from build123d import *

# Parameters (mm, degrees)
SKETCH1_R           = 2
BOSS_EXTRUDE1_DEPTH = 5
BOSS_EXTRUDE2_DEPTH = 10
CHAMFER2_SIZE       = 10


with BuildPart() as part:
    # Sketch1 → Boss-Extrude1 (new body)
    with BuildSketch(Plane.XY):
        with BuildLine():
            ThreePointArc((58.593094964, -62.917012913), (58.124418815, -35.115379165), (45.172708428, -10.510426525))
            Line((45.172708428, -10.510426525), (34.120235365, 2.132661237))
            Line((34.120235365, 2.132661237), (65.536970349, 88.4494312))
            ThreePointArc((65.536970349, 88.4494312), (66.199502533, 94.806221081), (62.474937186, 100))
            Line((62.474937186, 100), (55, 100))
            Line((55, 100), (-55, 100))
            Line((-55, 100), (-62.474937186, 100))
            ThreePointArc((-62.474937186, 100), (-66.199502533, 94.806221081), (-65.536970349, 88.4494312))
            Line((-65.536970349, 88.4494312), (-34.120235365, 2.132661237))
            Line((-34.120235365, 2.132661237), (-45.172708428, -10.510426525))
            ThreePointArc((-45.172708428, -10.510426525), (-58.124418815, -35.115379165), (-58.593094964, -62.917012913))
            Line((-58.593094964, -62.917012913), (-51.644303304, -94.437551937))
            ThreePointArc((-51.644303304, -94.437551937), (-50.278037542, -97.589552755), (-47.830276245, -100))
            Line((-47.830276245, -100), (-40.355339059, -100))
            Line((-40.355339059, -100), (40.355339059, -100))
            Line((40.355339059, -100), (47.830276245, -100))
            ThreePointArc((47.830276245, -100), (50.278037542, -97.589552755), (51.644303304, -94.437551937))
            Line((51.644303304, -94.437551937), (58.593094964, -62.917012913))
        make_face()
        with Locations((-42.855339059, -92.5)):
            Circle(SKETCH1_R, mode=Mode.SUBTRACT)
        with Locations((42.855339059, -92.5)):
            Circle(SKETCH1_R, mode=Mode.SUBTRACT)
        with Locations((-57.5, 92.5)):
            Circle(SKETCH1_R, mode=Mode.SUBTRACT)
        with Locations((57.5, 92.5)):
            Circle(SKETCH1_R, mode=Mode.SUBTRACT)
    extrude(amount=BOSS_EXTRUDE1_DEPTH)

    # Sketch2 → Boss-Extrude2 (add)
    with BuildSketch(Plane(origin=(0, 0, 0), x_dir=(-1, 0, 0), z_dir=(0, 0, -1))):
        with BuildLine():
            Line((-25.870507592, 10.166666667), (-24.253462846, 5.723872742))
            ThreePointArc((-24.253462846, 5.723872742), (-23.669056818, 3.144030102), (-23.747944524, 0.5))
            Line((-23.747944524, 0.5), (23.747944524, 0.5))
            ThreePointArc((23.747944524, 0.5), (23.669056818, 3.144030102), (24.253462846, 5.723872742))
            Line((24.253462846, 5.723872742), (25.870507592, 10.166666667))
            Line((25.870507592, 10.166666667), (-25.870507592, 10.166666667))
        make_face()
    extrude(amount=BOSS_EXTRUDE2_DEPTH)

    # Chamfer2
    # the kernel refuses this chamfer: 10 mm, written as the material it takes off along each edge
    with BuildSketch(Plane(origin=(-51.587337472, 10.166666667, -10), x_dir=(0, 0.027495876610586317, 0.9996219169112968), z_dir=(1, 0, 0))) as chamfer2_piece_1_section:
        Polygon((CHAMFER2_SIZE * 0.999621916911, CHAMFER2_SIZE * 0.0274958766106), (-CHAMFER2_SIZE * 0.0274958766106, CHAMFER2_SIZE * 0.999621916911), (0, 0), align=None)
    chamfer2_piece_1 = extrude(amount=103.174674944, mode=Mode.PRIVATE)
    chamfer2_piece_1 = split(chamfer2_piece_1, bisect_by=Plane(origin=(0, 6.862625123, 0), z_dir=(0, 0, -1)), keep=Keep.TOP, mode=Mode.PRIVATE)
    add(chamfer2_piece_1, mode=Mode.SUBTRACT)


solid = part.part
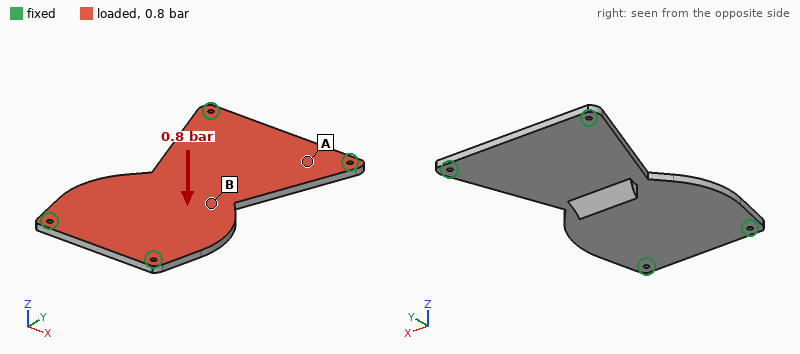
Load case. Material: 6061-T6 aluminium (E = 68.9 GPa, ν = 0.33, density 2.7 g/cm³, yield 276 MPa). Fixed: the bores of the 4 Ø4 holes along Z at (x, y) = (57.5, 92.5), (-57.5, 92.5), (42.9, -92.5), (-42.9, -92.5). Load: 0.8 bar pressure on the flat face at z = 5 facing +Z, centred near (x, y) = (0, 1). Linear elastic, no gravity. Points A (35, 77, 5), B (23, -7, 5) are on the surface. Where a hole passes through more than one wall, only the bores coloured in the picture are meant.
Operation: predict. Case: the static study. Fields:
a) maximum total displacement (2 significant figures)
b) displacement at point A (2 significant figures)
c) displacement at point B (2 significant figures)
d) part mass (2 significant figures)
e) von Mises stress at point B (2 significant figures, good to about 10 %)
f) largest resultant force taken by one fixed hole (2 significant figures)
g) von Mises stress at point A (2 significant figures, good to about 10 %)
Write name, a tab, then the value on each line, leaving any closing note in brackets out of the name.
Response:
maximum total displacement	0.54 mm
displacement at point A	0.14 mm
displacement at point B	0.52 mm
part mass	290 g
von Mises stress at point B	35 MPa
largest resultant force taken by one fixed hole	430 N
von Mises stress at point A	17 MPa
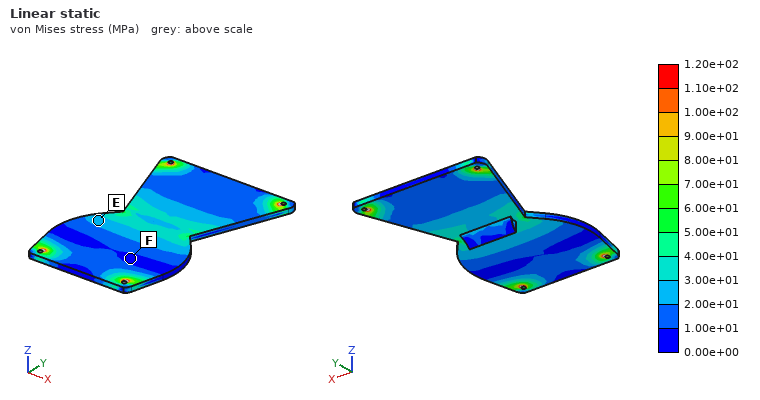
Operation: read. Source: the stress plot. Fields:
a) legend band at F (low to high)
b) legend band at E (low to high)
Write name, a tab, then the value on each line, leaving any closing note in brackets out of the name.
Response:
legend band at F	0.00e+00 to 1.00e+01 MPa
legend band at E	2.00e+01 to 3.00e+01 MPa
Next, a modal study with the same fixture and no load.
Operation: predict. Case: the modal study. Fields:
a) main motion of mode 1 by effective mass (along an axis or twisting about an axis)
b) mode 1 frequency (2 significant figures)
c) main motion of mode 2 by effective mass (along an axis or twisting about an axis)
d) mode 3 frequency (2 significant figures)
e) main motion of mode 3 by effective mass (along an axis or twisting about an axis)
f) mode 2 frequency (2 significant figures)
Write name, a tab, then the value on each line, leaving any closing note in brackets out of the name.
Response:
main motion of mode 1 by effective mass	along Z
mode 1 frequency	600 Hz
main motion of mode 2 by effective mass	twisting about Y
mode 3 frequency	1500 Hz
main motion of mode 3 by effective mass	twisting about X
mode 2 frequency	1300 Hz
